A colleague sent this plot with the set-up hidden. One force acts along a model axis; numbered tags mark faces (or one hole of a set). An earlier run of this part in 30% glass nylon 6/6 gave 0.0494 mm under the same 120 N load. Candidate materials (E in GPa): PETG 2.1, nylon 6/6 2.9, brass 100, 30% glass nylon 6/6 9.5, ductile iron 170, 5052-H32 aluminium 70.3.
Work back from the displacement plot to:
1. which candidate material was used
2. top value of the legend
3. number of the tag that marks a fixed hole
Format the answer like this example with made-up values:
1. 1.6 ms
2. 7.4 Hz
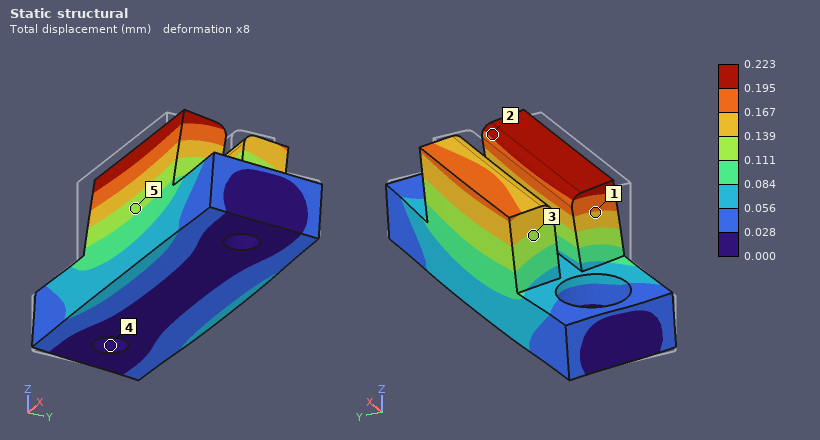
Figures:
1. PETG
2. 0.223 mm
3. 4
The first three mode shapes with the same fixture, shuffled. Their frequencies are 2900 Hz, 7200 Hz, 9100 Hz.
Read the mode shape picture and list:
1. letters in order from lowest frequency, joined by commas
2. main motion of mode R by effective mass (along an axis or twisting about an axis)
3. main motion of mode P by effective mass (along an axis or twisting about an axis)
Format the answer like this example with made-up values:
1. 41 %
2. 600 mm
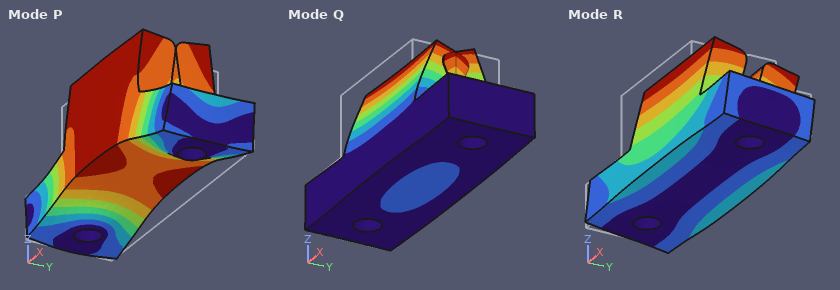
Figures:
1. R, P, Q
2. along Y
3. along Z
